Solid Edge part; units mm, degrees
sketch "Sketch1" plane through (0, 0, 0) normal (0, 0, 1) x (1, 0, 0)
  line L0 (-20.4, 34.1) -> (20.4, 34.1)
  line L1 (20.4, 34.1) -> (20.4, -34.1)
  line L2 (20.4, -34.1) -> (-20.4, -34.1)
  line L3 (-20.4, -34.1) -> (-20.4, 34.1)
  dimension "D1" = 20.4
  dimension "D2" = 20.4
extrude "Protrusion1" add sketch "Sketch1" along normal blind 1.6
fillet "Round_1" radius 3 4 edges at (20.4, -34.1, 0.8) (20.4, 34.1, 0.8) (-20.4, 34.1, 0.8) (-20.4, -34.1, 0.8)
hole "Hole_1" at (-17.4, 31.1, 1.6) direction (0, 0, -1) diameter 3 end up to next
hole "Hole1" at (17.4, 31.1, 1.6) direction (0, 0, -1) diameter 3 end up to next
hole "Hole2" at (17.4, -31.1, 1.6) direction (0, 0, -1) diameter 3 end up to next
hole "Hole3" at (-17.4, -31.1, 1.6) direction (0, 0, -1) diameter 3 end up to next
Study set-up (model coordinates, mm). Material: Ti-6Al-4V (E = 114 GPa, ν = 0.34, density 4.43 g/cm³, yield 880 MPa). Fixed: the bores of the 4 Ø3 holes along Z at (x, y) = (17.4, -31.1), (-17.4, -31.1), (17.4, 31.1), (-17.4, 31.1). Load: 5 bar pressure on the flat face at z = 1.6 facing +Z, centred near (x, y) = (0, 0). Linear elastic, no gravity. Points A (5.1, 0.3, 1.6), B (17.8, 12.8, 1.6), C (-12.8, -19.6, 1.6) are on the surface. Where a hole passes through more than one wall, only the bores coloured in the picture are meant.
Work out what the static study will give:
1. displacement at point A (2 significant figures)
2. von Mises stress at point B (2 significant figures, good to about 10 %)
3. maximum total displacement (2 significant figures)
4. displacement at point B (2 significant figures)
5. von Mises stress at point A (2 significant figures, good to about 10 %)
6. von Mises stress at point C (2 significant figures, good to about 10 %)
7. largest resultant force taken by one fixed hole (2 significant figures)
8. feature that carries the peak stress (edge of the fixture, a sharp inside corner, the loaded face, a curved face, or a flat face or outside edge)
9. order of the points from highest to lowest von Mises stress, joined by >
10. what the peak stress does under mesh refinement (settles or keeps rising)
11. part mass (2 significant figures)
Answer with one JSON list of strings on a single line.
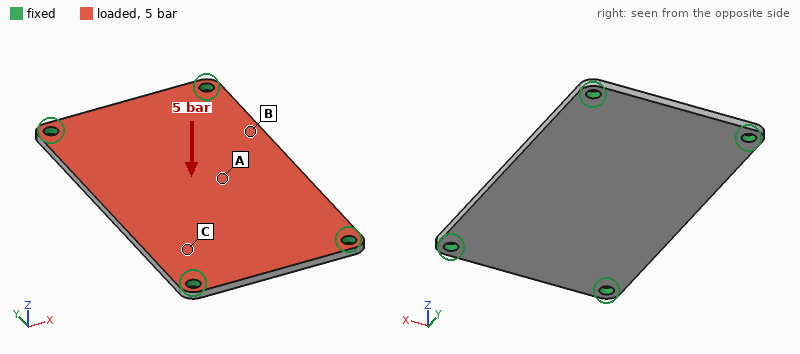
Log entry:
["0.64 mm", "140 MPa", "0.64 mm", "0.44 mm", "190 MPa", "58 MPa", "340 N", "edge of the fixture", "A > B > C", "keeps rising", "19 g"]
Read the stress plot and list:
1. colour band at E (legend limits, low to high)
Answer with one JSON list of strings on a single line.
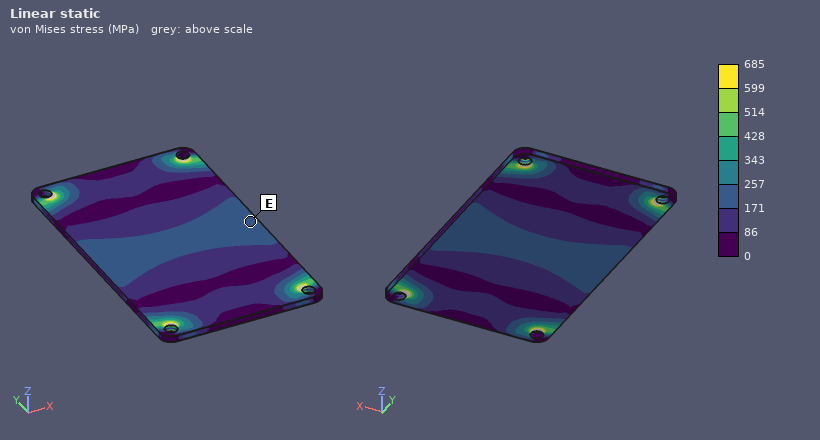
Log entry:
["171 to 257 MPa"]
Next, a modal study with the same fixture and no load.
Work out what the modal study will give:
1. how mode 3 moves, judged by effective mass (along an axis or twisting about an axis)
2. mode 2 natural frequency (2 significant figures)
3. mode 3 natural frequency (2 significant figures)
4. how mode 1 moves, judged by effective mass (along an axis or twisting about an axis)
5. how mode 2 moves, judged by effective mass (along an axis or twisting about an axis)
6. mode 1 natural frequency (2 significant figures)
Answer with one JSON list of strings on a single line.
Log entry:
["twisting about X", "3100 Hz", "5100 Hz", "along Z", "twisting about Y", "1900 Hz"]
